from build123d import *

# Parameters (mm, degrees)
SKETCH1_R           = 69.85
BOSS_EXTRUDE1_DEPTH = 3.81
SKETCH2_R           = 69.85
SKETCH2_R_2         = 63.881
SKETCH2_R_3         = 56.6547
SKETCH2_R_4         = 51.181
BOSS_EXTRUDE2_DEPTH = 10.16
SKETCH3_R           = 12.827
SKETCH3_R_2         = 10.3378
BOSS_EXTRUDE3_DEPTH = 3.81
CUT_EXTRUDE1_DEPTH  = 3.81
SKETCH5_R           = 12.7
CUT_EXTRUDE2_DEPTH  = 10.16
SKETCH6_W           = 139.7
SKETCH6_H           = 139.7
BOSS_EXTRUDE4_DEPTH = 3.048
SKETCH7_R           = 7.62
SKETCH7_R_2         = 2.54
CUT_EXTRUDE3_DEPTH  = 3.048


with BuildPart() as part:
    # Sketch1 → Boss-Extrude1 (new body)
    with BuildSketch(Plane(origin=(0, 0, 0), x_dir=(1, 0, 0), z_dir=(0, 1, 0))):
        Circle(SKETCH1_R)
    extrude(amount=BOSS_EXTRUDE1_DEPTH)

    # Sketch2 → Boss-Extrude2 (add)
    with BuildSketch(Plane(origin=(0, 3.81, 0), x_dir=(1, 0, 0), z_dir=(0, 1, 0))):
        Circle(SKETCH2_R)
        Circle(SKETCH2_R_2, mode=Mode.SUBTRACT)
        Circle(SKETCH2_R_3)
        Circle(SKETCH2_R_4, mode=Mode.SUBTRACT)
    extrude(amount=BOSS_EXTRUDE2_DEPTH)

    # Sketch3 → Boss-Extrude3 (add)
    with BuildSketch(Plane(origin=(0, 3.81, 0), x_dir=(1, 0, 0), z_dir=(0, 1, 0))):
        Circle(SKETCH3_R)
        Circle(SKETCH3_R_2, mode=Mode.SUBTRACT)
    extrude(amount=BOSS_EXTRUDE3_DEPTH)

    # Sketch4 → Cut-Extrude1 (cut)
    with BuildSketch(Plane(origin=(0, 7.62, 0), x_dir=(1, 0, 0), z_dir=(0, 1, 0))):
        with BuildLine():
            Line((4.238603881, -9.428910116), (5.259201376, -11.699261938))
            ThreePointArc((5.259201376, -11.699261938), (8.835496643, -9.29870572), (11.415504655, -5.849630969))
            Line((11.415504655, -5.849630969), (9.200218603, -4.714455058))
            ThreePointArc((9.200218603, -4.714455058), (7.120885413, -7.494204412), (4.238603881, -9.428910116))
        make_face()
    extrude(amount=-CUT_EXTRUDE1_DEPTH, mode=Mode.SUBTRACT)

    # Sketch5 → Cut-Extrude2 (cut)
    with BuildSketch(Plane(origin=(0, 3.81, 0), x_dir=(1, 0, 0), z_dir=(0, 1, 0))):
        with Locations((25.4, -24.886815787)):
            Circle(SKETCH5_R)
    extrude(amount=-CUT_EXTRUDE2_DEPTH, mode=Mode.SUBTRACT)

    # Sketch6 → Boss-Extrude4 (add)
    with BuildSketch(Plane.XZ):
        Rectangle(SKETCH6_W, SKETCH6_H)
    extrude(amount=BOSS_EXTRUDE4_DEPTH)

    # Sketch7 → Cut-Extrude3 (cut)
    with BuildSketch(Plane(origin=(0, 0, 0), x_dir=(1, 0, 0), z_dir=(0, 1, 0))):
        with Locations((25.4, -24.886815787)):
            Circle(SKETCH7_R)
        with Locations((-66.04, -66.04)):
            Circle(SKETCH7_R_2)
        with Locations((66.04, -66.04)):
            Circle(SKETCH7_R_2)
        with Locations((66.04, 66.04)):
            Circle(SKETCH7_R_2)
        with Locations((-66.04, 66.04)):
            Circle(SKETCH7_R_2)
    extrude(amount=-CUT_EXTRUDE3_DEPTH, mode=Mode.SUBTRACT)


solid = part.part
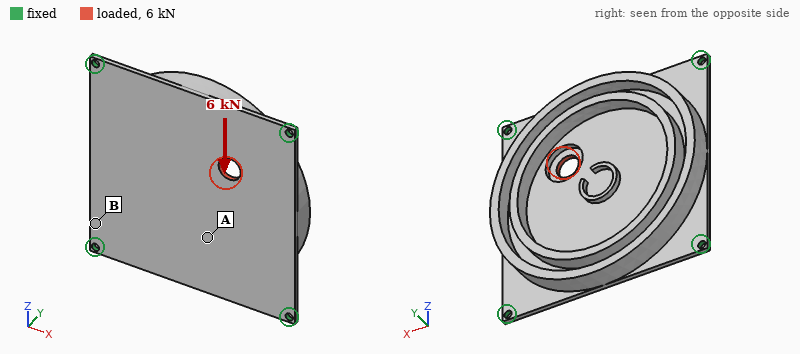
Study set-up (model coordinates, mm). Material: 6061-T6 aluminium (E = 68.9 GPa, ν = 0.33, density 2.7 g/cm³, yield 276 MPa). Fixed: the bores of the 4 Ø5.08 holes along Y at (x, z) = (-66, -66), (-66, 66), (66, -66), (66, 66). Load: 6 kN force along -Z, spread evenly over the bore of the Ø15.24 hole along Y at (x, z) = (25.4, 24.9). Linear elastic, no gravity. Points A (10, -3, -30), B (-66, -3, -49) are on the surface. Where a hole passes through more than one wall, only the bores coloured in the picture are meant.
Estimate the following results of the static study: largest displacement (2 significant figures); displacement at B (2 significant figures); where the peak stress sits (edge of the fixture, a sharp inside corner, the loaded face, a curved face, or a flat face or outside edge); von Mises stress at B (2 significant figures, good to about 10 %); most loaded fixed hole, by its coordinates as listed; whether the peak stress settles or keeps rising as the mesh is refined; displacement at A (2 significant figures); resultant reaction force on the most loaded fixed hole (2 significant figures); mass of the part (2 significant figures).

32 µm
5.3 µm
edge of the fixture
14 MPa
(66, 66)
keeps rising
20 µm
2.1 kN
430 g
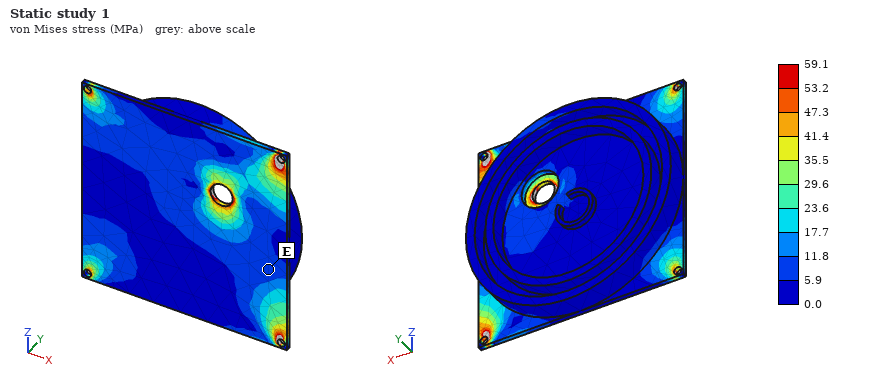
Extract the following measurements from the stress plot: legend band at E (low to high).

5.9 to 11.8 MPa
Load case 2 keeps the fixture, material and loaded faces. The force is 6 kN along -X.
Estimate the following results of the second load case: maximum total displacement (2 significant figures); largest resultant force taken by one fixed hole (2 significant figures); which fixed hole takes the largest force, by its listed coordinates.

32 µm
2.1 kN
(66, 66)
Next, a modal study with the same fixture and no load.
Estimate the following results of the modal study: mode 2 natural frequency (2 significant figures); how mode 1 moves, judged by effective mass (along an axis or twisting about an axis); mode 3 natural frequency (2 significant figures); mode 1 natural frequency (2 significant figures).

1200 Hz
along Y
1300 Hz
830 Hz
